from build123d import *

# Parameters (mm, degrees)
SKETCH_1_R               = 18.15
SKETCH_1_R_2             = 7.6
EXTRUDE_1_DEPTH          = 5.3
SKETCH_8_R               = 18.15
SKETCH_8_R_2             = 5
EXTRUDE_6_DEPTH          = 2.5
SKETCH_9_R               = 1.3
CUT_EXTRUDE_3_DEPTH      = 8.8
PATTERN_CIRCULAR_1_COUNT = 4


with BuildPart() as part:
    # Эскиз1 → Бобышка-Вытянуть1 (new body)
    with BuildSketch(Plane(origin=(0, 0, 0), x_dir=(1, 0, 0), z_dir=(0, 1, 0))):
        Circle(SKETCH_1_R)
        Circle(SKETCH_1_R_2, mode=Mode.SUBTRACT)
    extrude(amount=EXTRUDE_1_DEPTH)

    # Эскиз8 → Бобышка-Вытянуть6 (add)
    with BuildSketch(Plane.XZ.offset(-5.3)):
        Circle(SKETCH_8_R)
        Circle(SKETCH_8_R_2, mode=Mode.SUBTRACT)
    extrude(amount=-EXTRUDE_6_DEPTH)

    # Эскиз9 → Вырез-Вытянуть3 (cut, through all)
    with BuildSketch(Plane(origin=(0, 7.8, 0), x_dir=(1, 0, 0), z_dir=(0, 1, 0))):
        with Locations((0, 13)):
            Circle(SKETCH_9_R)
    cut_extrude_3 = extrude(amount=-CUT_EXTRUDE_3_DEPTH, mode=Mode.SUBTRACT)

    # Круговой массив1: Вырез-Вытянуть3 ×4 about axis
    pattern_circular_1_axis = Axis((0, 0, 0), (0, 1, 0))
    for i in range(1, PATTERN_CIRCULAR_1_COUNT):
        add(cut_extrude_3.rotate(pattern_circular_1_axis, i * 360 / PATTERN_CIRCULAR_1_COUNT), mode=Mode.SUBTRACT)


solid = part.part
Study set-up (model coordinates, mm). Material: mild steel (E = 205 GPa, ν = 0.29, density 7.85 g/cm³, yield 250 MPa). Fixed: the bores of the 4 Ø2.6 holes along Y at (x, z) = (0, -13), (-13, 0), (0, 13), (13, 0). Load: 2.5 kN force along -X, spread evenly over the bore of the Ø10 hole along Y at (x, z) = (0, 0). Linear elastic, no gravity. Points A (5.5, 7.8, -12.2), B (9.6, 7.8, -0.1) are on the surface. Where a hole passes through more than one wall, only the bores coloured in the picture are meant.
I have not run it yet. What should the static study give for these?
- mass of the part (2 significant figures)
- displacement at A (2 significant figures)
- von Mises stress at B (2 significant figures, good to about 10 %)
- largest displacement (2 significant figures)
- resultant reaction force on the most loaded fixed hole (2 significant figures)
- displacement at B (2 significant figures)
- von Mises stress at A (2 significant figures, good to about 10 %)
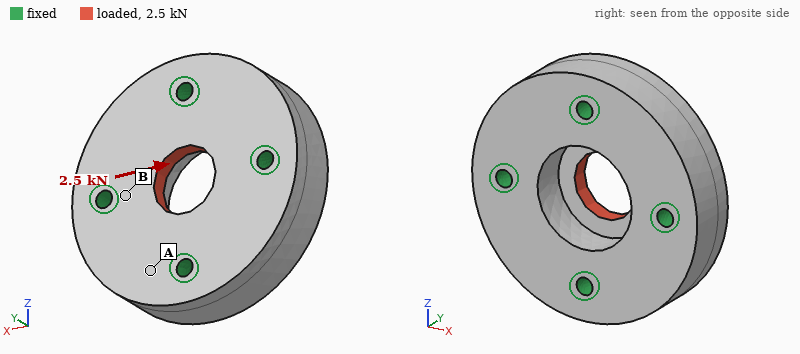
53 g
0.33 µm
39 MPa
1.4 µm
740 N
0.48 µm
8.3 MPa
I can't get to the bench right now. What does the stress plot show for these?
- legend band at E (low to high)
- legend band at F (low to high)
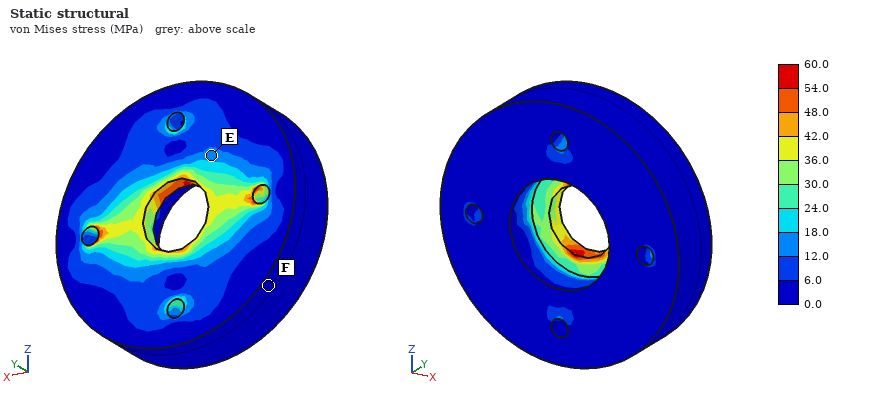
12.0 to 18.0 MPa
0.0 to 6.0 MPa
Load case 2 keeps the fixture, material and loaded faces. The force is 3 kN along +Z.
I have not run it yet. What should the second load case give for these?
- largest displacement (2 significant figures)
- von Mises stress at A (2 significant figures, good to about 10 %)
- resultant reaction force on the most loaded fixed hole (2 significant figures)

1.7 µm
11 MPa
890 N
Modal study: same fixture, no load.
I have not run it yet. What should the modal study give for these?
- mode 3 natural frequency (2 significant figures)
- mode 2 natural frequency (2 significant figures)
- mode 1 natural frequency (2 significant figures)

48 kHz
48 kHz
45 kHz
